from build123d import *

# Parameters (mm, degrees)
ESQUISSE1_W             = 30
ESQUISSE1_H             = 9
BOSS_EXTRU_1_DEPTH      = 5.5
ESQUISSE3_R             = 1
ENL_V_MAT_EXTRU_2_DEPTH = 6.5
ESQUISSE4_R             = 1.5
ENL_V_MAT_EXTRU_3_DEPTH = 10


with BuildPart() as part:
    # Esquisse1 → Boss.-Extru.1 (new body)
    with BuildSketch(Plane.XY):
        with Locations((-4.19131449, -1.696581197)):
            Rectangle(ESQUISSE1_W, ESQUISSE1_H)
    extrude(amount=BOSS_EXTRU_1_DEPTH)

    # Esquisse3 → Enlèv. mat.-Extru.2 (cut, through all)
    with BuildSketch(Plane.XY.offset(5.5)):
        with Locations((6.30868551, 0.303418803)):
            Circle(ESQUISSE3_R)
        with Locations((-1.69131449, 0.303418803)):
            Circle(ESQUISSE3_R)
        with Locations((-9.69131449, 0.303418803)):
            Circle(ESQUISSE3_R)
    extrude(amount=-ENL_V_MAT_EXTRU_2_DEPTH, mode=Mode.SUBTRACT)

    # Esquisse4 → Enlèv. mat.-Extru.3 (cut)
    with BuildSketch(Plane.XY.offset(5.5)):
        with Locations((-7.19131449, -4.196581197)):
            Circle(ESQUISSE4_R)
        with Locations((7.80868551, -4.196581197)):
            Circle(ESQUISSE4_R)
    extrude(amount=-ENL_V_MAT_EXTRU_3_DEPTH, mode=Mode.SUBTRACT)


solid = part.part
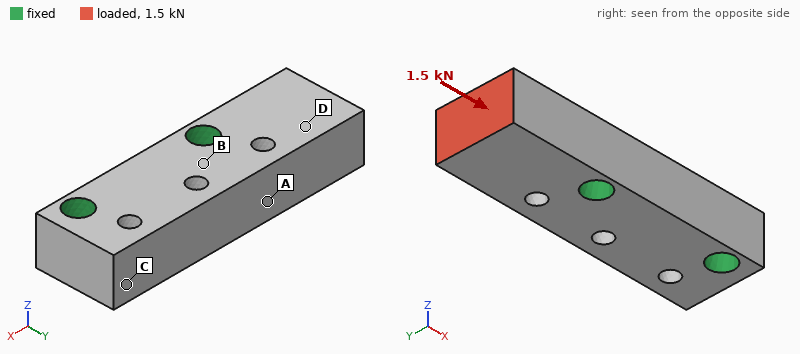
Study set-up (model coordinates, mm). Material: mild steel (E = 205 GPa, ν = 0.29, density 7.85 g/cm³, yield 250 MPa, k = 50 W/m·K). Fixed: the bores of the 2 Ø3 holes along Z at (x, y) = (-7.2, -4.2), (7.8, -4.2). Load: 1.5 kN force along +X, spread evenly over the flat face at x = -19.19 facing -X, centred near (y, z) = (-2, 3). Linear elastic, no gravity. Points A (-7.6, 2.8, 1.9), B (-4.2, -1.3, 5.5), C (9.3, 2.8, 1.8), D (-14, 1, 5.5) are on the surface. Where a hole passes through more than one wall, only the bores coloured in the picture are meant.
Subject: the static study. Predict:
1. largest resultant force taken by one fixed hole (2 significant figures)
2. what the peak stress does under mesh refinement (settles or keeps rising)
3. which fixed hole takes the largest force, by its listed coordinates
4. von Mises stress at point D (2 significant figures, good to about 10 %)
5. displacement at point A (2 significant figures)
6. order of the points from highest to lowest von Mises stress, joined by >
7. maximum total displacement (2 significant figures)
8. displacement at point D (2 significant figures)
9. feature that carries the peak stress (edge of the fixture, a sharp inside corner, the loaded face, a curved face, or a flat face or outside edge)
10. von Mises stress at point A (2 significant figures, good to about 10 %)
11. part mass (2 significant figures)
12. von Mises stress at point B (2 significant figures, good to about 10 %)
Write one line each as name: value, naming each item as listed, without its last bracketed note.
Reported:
largest resultant force taken by one fixed hole: 1.3 kN
what the peak stress does under mesh refinement: keeps rising
which fixed hole takes the largest force, by its listed coordinates: (-7.2, -4.2)
von Mises stress at point D: 28 MPa
displacement at point A: 1.5 µm
order of the points from highest to lowest von Mises stress, joined by >: A > D > B > C
maximum total displacement: 4.5 µm
displacement at point D: 2.7 µm
feature that carries the peak stress: edge of the fixture
von Mises stress at point A: 42 MPa
part mass: 11 g
von Mises stress at point B: 16 MPa
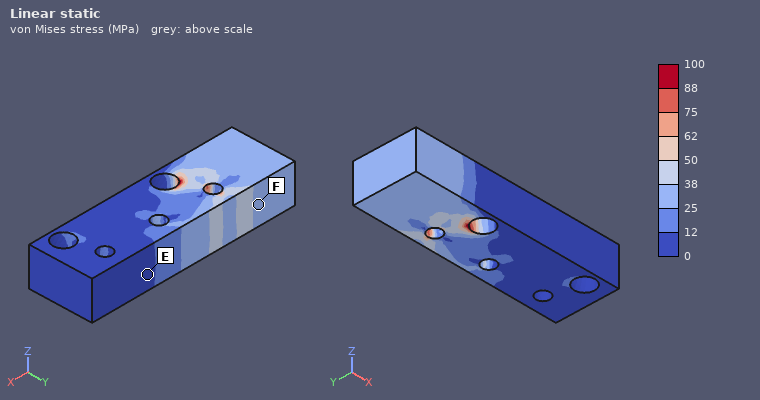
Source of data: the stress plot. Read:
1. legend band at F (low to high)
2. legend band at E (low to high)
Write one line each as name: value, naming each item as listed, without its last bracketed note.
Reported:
legend band at F: 25 to 38 MPa
legend band at E: 0 to 12 MPa
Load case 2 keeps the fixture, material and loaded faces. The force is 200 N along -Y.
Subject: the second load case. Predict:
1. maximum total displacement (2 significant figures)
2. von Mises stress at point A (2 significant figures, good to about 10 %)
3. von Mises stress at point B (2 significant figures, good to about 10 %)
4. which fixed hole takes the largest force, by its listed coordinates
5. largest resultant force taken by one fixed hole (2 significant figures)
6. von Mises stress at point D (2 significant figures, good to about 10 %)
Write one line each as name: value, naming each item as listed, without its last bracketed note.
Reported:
maximum total displacement: 3.9 µm
von Mises stress at point A: 28 MPa
von Mises stress at point B: 7.6 MPa
which fixed hole takes the largest force, by its listed coordinates: (-7.2, -4.2)
largest resultant force taken by one fixed hole: 310 N
von Mises stress at point D: 11 MPa
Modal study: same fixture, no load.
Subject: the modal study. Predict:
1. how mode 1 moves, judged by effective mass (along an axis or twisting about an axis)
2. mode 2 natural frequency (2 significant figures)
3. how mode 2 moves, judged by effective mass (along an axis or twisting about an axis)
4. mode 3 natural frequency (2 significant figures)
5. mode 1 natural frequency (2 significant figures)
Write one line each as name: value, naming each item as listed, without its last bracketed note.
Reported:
how mode 1 moves, judged by effective mass: along Z
mode 2 natural frequency: 31 kHz
how mode 2 moves, judged by effective mass: along Y
mode 3 natural frequency: 49 kHz
mode 1 natural frequency: 26 kHz
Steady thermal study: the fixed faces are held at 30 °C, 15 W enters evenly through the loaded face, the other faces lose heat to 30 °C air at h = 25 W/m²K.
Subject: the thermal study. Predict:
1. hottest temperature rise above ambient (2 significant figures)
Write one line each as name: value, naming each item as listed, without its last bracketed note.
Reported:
hottest temperature rise above ambient: 75 K
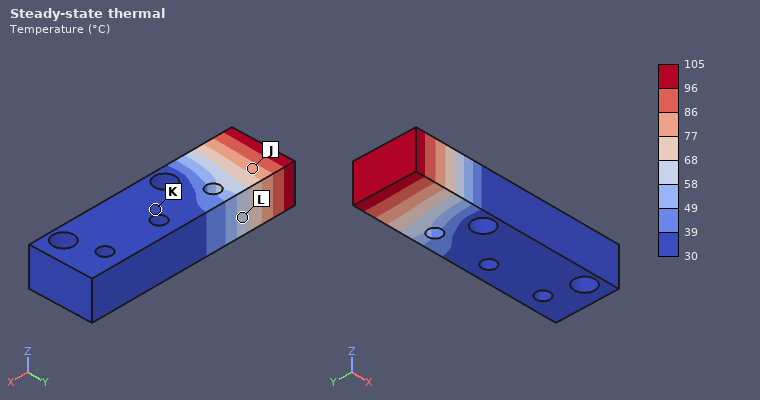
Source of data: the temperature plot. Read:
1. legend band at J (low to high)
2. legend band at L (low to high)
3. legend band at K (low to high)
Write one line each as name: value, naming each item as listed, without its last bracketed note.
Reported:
legend band at J: 77 to 86 °C
legend band at L: 58 to 68 °C
legend band at K: 30 to 39 °C
